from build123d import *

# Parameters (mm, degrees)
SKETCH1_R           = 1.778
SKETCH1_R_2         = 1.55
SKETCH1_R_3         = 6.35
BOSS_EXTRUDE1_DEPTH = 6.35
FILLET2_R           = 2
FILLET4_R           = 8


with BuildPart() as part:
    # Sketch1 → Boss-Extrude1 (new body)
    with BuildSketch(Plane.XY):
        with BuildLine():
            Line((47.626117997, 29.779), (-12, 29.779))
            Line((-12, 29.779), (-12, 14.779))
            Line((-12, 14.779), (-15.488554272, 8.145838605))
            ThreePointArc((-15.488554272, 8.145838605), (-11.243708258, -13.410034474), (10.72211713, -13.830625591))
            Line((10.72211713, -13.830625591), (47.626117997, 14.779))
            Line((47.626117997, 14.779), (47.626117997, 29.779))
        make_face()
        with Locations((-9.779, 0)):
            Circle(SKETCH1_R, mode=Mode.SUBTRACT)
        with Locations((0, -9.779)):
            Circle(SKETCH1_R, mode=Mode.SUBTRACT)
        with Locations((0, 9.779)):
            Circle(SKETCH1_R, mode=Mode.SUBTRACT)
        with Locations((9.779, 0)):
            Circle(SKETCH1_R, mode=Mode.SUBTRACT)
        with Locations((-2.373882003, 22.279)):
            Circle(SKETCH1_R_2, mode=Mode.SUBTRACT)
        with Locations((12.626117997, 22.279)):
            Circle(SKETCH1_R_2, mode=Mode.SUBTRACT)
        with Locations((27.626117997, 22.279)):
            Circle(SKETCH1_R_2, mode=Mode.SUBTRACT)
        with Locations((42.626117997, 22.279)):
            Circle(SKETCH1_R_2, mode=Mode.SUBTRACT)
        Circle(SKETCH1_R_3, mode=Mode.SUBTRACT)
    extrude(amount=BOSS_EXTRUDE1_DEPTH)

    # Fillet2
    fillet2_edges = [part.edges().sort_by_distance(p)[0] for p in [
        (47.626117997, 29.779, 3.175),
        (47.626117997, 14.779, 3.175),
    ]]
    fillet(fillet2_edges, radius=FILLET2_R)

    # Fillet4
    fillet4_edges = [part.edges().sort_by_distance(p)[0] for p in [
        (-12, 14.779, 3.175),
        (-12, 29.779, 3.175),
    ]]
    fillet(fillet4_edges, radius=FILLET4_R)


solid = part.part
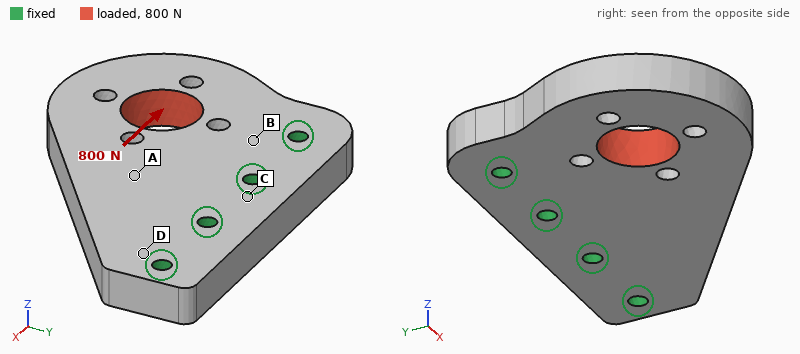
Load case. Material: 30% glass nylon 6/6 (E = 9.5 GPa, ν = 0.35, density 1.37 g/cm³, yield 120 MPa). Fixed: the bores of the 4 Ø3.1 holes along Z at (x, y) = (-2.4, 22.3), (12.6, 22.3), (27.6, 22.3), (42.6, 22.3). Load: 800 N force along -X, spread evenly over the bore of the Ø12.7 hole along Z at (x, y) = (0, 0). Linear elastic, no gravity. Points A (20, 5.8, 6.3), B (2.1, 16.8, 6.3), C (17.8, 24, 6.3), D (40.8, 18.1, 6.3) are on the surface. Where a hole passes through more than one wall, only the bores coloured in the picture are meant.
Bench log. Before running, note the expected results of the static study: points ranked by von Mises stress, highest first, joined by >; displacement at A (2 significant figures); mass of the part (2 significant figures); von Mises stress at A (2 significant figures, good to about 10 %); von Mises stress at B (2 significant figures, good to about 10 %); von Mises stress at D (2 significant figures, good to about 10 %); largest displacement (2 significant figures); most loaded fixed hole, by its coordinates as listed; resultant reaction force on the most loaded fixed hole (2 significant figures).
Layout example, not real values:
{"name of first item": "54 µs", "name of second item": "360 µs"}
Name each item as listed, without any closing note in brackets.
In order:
{"points ranked by von Mises stress, highest first, joined by >": "B > D > A > C", "displacement at A": "14 µm", "mass of the part": "18 g", "von Mises stress at A": "4.1 MPa", "von Mises stress at B": "8.6 MPa", "von Mises stress at D": "5.9 MPa", "largest displacement": "51 µm", "most loaded fixed hole, by its coordinates as listed": "(-2.4, 22.3)", "resultant reaction force on the most loaded fixed hole": "490 N"}
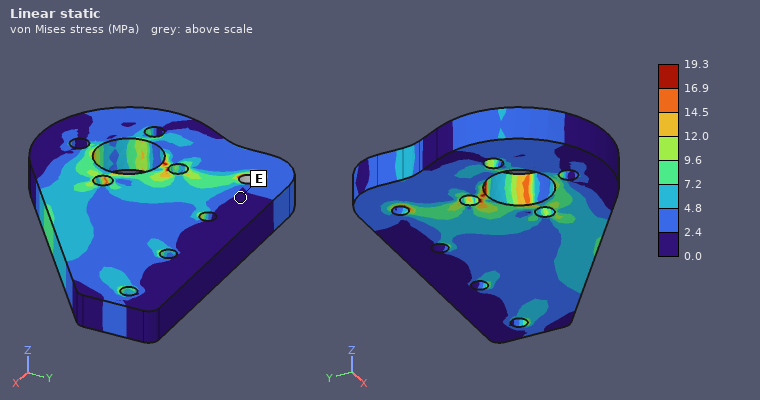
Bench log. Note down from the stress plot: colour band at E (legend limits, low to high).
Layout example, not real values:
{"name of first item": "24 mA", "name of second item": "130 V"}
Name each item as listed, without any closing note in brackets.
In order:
{"colour band at E": "0.0 to 2.4 MPa"}
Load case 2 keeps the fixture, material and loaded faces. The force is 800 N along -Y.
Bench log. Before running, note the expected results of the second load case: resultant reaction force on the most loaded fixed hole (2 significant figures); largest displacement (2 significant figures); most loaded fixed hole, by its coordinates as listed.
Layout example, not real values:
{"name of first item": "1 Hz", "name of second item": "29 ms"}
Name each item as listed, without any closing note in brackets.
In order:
{"resultant reaction force on the most loaded fixed hole": "600 N", "largest displacement": "31 µm", "most loaded fixed hole, by its coordinates as listed": "(-2.4, 22.3)"}
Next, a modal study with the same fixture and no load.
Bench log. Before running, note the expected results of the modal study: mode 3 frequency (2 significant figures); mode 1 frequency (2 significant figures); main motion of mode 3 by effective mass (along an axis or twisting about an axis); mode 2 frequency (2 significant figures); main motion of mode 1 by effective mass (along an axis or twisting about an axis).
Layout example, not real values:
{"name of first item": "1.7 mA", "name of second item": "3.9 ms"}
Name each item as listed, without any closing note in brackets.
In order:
{"mode 3 frequency": "7800 Hz", "mode 1 frequency": "2000 Hz", "main motion of mode 3 by effective mass": "along X", "mode 2 frequency": "4600 Hz", "main motion of mode 1 by effective mass": "along Z"}
